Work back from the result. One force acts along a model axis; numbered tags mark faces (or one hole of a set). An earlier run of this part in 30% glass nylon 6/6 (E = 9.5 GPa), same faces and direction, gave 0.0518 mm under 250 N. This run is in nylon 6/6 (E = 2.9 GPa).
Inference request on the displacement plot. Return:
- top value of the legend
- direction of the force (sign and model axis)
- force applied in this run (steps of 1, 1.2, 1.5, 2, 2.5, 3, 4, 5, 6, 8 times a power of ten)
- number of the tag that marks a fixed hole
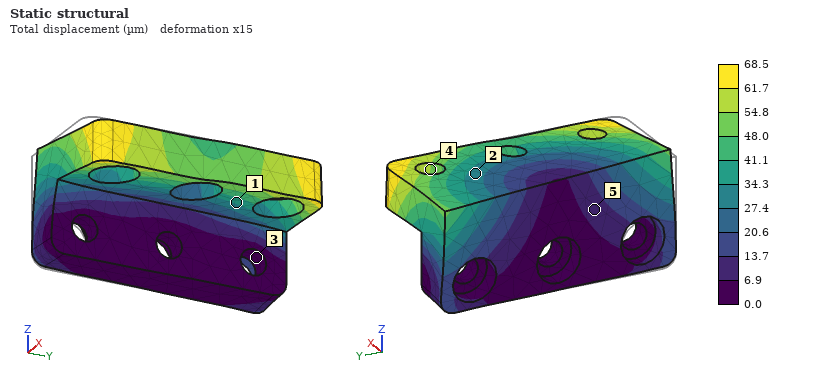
68.5 µm
+Y
100 N
3
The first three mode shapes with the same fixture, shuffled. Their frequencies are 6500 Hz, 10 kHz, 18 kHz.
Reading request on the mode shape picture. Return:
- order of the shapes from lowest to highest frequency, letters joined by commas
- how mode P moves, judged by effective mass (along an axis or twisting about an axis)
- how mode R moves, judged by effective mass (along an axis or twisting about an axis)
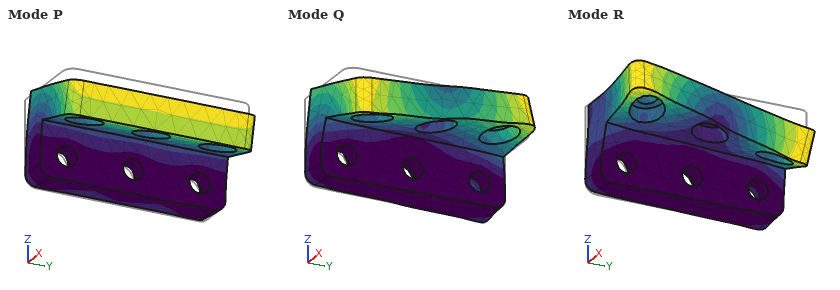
P, Q, R
along X
along Y
